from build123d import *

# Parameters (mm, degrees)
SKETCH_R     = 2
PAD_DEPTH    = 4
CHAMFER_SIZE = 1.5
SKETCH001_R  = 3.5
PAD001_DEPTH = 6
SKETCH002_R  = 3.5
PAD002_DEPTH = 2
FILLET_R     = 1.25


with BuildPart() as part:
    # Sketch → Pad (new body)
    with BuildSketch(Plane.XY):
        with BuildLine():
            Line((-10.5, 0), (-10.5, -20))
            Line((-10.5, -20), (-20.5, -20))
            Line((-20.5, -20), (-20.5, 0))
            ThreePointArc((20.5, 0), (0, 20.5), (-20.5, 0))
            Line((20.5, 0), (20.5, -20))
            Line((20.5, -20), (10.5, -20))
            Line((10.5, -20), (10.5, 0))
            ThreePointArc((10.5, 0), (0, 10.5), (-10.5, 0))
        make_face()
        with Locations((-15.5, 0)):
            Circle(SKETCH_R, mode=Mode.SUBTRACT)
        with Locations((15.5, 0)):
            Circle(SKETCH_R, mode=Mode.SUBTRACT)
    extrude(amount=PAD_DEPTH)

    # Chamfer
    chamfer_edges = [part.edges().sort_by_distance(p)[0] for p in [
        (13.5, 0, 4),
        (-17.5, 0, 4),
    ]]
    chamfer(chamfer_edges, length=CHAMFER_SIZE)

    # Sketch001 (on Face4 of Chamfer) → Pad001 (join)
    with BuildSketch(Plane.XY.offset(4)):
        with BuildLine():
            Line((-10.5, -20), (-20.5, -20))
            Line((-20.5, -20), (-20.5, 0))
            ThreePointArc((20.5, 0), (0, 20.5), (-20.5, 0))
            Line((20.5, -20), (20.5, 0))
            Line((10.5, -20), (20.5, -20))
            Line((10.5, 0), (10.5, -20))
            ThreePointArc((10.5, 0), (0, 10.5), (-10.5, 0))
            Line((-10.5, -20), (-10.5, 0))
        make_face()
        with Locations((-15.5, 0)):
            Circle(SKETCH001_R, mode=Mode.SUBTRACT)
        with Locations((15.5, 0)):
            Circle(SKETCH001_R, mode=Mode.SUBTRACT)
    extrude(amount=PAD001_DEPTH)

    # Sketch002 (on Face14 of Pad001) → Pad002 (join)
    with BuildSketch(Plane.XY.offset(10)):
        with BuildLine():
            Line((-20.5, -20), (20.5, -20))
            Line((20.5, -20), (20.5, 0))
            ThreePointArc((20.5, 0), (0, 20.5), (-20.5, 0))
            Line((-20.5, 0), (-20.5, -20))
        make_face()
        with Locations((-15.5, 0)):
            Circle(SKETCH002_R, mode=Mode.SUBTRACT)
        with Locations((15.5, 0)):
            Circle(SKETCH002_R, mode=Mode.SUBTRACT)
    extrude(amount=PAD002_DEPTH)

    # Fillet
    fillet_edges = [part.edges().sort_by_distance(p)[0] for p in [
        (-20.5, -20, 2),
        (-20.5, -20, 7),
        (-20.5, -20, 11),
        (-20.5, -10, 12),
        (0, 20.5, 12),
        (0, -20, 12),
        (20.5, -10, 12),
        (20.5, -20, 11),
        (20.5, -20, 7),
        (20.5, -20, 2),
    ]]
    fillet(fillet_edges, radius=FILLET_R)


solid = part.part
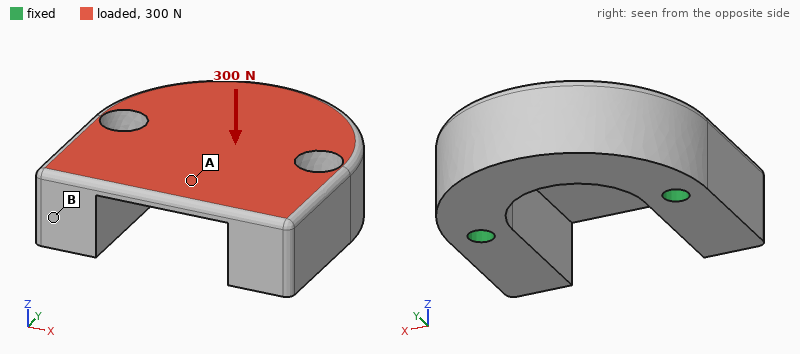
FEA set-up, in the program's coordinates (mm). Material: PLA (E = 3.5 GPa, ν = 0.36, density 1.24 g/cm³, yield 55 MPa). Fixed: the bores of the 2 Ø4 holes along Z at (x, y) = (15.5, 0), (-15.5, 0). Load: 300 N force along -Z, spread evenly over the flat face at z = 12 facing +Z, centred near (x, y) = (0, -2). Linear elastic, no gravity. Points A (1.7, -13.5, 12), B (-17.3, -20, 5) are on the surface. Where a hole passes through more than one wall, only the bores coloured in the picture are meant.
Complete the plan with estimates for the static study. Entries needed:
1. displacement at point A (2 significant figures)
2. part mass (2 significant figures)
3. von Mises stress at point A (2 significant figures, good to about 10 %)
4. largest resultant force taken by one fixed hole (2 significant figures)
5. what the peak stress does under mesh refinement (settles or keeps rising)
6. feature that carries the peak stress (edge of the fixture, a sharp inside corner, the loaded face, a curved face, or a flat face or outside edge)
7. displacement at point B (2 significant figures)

0.13 mm
14 g
7.3 MPa
160 N
keeps rising
edge of the fixture
0.067 mm
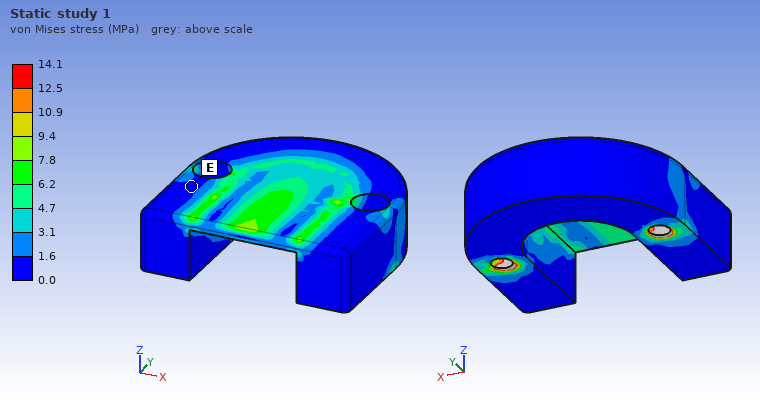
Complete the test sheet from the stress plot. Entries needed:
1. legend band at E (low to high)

0.0 to 1.6 MPa
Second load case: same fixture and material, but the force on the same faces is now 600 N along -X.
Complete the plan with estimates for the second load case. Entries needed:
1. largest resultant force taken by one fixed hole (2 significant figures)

330 N
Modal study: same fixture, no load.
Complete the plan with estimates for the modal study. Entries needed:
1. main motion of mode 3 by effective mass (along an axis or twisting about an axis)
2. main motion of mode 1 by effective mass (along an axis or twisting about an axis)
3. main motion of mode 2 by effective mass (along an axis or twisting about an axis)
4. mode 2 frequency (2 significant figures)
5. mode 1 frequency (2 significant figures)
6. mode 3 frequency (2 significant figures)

along Z
along Y
along X
2900 Hz
1500 Hz
4900 Hz
